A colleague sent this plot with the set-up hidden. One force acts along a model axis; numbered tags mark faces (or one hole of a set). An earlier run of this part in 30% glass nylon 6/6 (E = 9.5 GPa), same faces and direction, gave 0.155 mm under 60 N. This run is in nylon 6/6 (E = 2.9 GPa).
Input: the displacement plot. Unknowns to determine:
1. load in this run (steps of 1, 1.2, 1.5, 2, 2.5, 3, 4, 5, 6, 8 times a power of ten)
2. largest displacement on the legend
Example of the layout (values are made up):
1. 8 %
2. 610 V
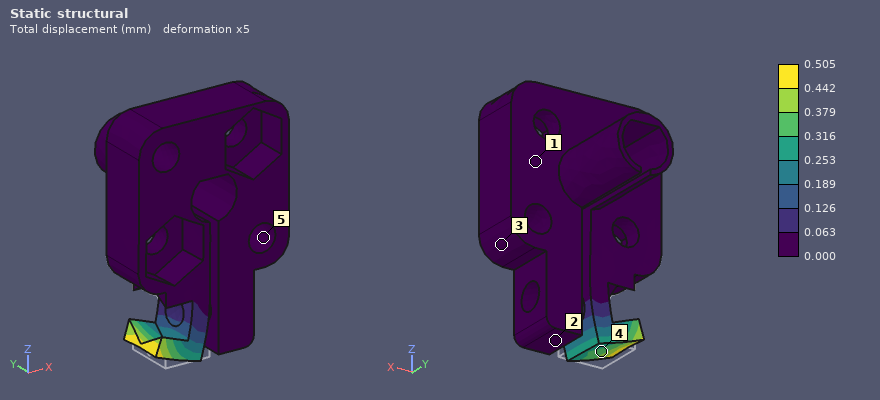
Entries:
1. 60 N
2. 0.505 mm
